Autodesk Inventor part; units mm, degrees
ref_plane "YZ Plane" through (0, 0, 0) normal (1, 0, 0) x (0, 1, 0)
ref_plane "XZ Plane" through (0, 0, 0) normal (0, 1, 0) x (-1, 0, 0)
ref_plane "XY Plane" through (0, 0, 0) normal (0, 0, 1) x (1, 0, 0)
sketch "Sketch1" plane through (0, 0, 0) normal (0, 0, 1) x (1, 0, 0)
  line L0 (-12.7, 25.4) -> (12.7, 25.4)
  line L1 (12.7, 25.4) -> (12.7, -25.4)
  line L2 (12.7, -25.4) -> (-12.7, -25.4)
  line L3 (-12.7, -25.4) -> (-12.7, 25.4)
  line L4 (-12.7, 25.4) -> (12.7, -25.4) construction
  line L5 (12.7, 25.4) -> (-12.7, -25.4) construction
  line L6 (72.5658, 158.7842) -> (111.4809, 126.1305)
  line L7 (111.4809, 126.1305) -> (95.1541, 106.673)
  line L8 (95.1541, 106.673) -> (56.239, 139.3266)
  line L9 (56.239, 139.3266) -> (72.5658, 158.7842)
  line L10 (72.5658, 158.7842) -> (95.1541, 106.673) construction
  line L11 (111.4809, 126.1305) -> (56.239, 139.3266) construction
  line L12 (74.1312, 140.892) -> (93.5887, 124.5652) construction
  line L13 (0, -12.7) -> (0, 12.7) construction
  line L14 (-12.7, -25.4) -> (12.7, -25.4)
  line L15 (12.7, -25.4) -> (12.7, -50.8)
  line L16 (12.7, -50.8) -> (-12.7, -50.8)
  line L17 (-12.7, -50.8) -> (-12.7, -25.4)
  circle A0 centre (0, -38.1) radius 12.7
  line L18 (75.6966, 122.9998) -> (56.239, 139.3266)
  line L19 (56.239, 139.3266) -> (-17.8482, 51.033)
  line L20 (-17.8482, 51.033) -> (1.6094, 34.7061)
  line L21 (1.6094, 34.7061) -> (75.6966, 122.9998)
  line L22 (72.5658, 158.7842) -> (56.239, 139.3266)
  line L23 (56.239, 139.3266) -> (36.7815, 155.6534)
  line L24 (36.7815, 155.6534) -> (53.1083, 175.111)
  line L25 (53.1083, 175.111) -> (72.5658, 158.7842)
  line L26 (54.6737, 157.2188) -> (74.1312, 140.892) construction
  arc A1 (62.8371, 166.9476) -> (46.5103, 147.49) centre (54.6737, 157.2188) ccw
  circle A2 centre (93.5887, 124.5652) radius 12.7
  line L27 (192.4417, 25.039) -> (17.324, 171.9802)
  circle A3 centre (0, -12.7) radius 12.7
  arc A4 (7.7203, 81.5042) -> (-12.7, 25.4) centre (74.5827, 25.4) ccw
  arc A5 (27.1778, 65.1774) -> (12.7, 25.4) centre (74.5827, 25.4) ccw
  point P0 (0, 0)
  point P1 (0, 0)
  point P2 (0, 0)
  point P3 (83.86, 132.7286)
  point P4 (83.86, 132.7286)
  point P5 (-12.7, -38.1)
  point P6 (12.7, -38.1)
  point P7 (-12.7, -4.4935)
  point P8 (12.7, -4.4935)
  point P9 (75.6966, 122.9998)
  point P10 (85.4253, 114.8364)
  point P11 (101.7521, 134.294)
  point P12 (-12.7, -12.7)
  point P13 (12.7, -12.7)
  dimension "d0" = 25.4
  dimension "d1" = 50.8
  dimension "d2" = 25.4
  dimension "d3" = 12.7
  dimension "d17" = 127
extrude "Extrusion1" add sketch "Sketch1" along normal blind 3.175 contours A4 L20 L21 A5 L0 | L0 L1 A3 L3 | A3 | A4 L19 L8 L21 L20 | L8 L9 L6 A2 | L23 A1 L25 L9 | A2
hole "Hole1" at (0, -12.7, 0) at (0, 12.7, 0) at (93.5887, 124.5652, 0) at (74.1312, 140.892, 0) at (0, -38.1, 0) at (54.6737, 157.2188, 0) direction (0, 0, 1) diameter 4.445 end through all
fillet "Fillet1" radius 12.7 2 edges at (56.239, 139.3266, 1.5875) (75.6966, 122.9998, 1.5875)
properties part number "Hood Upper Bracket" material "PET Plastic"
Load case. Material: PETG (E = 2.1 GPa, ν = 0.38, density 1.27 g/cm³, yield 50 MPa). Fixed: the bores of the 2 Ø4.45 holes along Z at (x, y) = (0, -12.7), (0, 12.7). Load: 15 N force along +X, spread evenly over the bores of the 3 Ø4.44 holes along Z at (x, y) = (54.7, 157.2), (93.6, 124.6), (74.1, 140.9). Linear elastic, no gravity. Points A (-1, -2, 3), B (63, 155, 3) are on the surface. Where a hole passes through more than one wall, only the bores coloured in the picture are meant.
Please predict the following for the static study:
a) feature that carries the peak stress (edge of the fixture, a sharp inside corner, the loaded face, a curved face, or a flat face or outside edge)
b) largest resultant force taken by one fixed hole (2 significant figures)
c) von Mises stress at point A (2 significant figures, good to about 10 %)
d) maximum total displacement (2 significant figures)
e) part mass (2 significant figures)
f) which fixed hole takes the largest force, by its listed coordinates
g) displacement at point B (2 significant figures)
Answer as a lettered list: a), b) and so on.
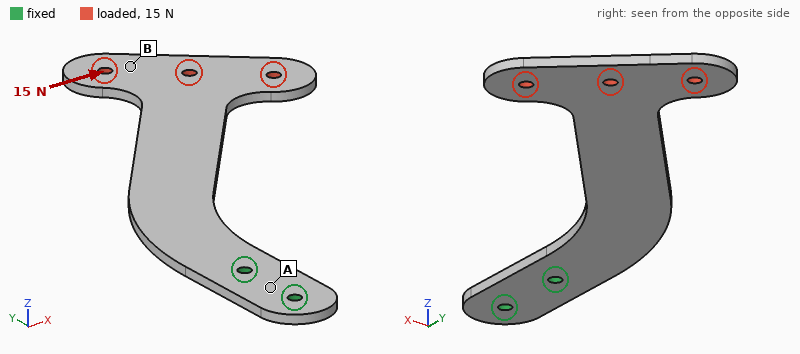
a) edge of the fixture
b) 73 N
c) 1.7 MPa
d) 2.3 mm
e) 25 g
f) (0, 12.7)
g) 2.1 mm
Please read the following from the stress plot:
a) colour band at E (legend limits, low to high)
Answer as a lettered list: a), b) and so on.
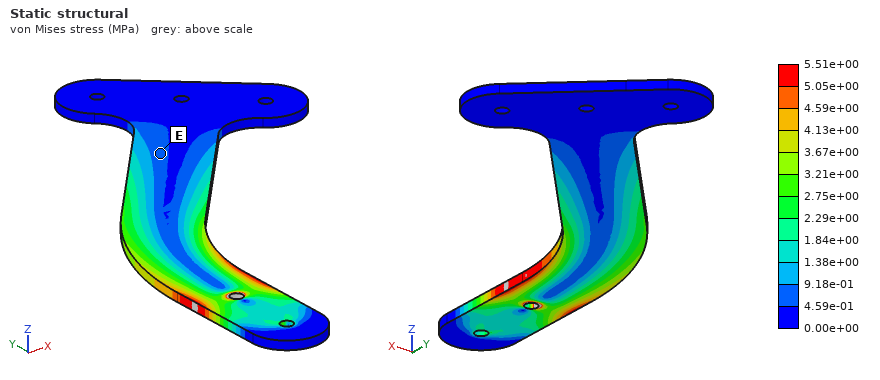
a) 4.59e-01 to 9.18e-01 MPa
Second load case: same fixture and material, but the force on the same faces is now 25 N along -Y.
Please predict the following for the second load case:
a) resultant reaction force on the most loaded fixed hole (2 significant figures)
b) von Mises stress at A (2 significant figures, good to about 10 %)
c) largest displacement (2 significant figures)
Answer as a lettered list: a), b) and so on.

a) 60 N
b) 1.6 MPa
c) 2.7 mm
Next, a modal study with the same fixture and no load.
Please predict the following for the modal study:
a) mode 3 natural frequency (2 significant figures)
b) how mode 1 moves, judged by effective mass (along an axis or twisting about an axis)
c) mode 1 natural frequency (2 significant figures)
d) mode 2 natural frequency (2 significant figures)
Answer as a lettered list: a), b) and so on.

a) 120 Hz
b) along Z
c) 18 Hz
d) 98 Hz
